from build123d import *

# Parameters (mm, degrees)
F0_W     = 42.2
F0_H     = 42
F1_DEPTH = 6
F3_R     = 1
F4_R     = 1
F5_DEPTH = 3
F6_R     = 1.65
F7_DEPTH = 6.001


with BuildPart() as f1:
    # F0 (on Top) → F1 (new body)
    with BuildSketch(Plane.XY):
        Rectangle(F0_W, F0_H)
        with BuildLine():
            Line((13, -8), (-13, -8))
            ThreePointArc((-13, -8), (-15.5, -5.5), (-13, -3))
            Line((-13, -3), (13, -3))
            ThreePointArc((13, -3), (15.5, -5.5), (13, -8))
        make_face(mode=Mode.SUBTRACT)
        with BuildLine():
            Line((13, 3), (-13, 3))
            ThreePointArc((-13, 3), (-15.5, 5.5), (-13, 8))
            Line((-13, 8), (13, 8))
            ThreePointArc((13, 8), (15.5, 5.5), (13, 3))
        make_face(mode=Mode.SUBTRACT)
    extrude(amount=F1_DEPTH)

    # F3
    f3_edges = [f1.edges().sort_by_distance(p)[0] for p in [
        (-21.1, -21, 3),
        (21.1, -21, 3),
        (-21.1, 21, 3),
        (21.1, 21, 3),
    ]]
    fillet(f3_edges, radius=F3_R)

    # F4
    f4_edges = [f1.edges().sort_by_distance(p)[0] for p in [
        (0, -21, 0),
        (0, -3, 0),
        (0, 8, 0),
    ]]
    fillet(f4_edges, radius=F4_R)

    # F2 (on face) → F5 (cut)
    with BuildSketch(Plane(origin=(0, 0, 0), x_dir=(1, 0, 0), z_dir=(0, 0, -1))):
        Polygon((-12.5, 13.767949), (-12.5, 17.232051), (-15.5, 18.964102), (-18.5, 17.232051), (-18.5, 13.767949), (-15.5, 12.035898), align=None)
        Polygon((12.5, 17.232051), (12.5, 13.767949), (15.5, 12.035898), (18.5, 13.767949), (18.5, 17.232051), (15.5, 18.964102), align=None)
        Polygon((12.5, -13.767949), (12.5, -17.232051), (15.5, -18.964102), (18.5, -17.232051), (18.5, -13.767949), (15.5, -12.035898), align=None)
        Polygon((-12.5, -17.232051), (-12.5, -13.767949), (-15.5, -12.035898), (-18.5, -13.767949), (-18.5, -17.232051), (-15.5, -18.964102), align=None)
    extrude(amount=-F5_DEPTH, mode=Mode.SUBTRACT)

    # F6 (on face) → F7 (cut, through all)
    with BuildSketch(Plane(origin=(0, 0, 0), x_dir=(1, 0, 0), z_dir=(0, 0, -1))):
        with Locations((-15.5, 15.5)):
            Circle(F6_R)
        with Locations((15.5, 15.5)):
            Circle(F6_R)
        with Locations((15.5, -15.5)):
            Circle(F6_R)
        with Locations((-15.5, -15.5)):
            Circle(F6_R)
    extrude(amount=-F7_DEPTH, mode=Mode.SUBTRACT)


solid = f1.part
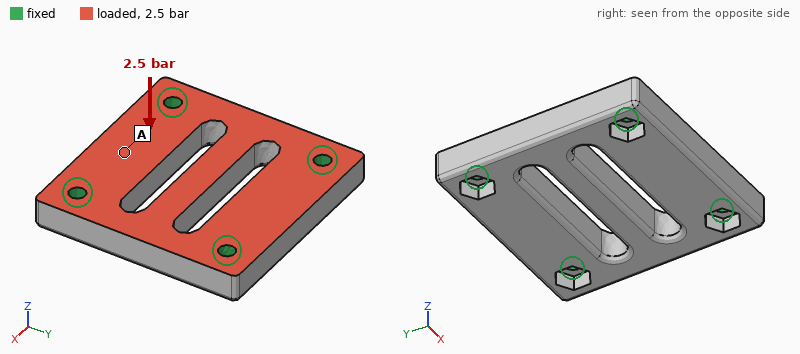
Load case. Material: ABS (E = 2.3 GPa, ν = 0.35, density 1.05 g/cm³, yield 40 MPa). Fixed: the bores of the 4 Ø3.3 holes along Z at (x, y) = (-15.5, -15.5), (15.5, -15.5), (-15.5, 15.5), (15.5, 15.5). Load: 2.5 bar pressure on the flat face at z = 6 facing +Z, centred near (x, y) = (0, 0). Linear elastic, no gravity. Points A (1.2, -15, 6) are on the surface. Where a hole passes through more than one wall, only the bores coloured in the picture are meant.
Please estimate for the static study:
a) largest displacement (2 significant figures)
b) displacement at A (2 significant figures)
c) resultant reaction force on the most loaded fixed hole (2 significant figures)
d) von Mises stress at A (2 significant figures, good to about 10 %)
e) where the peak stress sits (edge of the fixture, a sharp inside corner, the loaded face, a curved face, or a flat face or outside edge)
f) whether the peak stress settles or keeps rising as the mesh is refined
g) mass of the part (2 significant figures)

0.12 mm
0.036 mm
95 N
1.8 MPa
edge of the fixture
keeps rising
8.7 g
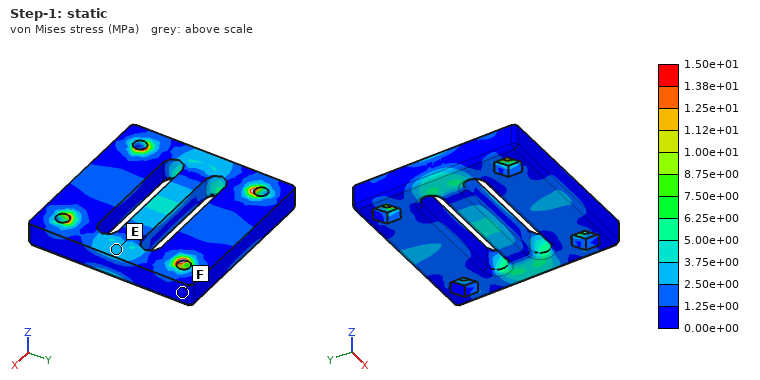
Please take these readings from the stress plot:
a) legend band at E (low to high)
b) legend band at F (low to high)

2.50e+00 to 3.75e+00 MPa
0.00e+00 to 1.25e+00 MPa
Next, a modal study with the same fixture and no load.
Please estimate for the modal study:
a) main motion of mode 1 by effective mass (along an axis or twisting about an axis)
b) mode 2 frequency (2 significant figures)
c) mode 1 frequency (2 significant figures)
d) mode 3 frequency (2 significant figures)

along Z
6000 Hz
3600 Hz
6000 Hz
